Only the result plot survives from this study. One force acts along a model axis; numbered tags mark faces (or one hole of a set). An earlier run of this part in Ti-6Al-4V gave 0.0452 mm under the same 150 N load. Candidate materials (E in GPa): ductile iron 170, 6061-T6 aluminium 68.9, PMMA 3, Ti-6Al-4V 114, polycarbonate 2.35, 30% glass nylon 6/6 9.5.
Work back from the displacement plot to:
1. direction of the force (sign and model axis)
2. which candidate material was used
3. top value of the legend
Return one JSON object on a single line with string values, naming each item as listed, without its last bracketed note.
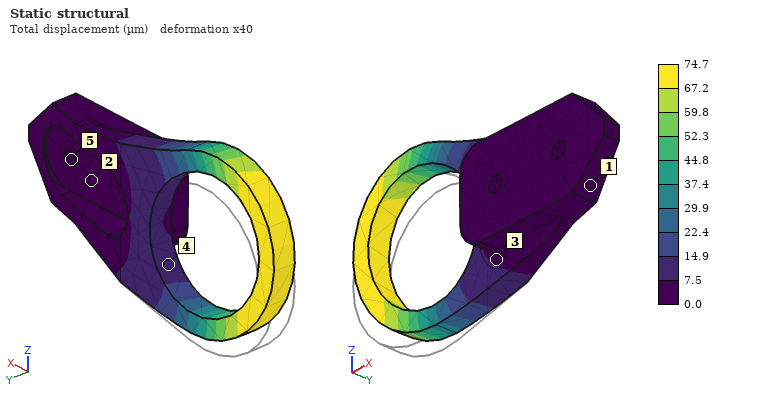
{"direction of the force": "+Z", "which candidate material was used": "6061-T6 aluminium", "top value of the legend": "74.7 µm"}
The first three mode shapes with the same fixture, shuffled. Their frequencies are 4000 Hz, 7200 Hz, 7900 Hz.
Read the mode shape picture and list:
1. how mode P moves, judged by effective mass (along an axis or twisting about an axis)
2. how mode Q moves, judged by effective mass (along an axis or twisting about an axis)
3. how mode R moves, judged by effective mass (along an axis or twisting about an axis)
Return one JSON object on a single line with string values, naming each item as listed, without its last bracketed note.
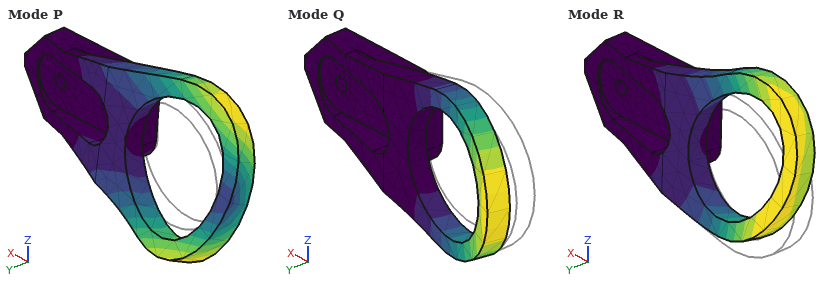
{"how mode P moves, judged by effective mass": "twisting about X", "how mode Q moves, judged by effective mass": "along Y", "how mode R moves, judged by effective mass": "along Z"}
